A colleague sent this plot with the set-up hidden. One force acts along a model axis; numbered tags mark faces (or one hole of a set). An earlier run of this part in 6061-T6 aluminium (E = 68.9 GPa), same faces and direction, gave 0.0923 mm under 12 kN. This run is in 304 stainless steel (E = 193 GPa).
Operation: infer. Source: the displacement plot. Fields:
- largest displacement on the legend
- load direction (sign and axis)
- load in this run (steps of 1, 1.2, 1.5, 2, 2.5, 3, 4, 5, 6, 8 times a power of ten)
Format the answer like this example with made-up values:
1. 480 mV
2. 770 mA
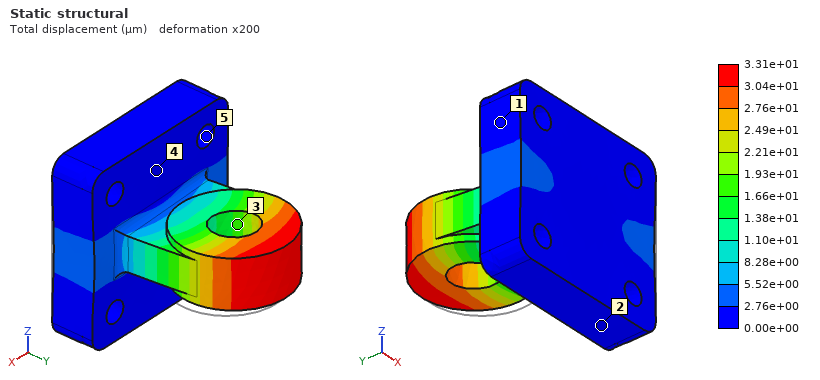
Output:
1. 3.31e+01 µm
2. -X
3. 12 kN
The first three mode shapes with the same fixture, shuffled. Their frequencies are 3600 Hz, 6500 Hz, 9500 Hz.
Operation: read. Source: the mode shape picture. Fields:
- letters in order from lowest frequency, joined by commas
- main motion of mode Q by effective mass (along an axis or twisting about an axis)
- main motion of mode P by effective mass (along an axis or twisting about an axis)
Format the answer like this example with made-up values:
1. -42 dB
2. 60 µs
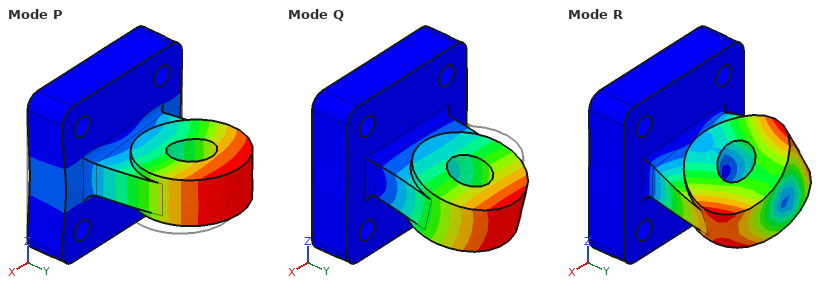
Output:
1. Q, P, R
2. along Z
3. along X
